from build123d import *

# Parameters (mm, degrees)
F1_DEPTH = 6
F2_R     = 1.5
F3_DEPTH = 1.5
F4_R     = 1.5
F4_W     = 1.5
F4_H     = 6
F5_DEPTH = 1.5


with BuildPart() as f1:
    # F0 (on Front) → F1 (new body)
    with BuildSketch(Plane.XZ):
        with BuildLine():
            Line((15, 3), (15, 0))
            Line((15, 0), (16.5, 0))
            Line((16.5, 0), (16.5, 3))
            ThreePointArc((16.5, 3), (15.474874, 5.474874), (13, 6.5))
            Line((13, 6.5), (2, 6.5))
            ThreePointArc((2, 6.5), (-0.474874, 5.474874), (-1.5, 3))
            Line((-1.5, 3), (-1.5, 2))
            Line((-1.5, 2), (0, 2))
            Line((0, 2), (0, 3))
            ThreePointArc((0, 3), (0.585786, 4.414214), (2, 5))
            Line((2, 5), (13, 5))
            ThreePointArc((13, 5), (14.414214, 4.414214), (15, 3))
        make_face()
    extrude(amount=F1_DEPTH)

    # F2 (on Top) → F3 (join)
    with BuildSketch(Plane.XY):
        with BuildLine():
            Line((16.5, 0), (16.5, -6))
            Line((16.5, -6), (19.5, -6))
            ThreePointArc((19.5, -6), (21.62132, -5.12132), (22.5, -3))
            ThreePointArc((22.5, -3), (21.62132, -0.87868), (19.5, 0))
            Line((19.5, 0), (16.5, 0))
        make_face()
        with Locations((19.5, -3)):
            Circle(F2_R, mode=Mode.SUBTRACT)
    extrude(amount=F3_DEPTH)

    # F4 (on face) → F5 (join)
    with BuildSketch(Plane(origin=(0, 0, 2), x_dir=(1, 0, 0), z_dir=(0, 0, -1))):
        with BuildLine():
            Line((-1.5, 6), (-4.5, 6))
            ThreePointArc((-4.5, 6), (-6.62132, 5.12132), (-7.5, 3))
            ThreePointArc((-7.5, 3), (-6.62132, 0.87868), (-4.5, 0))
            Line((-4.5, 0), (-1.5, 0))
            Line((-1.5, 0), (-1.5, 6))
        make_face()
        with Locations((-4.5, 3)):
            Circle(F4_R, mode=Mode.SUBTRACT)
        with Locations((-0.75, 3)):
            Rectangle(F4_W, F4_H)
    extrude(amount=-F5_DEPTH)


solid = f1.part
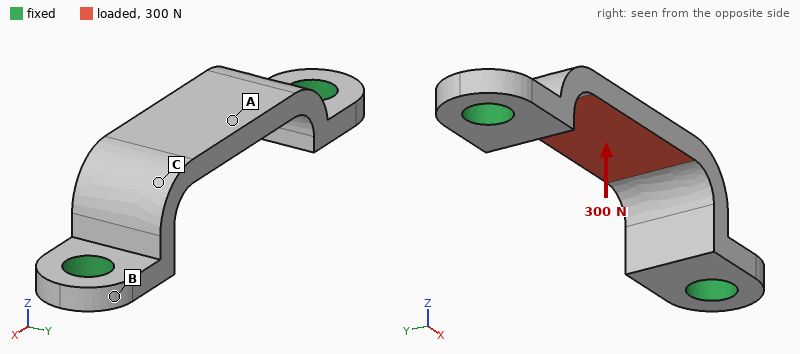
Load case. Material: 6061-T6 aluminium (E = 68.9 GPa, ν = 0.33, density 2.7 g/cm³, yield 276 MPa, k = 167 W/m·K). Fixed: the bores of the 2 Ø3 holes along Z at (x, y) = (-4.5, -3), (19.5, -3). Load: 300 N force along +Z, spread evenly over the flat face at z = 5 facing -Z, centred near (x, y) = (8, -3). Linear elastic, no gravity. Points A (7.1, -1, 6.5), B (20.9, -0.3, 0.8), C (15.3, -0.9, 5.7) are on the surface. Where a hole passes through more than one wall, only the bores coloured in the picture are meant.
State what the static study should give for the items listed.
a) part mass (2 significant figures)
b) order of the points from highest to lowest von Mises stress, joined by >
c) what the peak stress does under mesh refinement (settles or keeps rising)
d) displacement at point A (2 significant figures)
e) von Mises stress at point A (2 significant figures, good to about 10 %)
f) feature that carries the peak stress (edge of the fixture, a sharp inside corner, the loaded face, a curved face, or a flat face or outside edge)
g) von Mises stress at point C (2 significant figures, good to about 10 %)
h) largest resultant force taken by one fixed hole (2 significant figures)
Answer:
0.78 g
A > C > B
keeps rising
47 µm
150 MPa
edge of the fixture
97 MPa
250 N
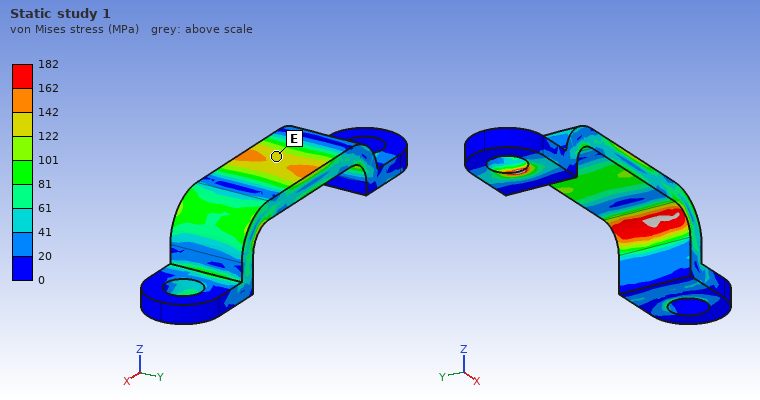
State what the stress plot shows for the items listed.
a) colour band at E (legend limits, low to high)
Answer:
122 to 142 MPa
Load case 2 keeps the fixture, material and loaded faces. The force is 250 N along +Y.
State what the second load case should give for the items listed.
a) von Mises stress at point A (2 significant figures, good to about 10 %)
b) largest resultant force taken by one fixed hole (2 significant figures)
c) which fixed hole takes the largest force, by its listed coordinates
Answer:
48 MPa
140 N
(-4.5, -3)
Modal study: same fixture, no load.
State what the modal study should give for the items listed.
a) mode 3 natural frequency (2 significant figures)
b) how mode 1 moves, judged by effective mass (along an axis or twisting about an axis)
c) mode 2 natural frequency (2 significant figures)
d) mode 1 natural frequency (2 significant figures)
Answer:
31 kHz
along Y
24 kHz
21 kHz
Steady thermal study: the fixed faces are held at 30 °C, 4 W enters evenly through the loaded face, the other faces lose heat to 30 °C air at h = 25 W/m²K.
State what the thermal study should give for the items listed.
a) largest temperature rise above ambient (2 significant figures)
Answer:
14 K
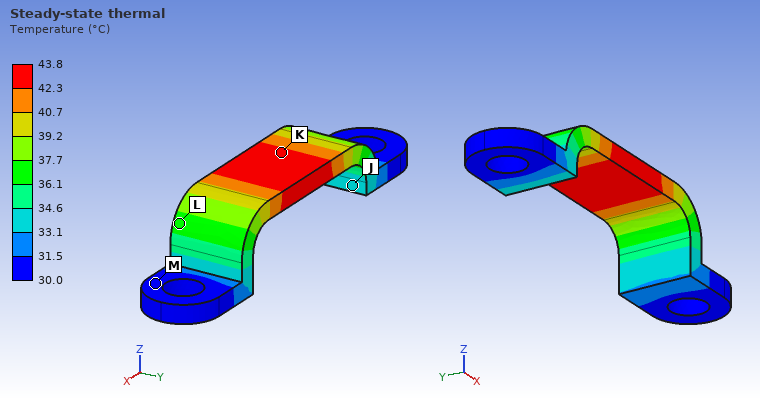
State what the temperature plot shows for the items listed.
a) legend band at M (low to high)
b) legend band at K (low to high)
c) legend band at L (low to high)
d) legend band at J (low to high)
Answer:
30.0 to 31.5 °C
42.3 to 43.8 °C
36.1 to 37.7 °C
33.1 to 34.6 °C
